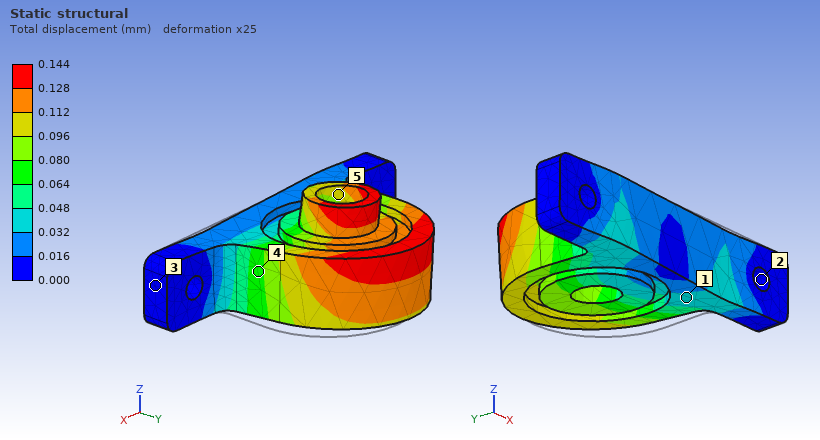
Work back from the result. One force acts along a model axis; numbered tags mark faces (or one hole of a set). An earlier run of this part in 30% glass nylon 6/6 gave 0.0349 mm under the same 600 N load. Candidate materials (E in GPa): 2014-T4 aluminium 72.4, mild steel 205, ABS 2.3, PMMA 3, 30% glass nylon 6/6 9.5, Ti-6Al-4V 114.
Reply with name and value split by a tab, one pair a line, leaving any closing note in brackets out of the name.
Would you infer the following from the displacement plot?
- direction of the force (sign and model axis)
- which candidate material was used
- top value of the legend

direction of the force	-X
which candidate material was used	ABS
top value of the legend	0.144 mm
